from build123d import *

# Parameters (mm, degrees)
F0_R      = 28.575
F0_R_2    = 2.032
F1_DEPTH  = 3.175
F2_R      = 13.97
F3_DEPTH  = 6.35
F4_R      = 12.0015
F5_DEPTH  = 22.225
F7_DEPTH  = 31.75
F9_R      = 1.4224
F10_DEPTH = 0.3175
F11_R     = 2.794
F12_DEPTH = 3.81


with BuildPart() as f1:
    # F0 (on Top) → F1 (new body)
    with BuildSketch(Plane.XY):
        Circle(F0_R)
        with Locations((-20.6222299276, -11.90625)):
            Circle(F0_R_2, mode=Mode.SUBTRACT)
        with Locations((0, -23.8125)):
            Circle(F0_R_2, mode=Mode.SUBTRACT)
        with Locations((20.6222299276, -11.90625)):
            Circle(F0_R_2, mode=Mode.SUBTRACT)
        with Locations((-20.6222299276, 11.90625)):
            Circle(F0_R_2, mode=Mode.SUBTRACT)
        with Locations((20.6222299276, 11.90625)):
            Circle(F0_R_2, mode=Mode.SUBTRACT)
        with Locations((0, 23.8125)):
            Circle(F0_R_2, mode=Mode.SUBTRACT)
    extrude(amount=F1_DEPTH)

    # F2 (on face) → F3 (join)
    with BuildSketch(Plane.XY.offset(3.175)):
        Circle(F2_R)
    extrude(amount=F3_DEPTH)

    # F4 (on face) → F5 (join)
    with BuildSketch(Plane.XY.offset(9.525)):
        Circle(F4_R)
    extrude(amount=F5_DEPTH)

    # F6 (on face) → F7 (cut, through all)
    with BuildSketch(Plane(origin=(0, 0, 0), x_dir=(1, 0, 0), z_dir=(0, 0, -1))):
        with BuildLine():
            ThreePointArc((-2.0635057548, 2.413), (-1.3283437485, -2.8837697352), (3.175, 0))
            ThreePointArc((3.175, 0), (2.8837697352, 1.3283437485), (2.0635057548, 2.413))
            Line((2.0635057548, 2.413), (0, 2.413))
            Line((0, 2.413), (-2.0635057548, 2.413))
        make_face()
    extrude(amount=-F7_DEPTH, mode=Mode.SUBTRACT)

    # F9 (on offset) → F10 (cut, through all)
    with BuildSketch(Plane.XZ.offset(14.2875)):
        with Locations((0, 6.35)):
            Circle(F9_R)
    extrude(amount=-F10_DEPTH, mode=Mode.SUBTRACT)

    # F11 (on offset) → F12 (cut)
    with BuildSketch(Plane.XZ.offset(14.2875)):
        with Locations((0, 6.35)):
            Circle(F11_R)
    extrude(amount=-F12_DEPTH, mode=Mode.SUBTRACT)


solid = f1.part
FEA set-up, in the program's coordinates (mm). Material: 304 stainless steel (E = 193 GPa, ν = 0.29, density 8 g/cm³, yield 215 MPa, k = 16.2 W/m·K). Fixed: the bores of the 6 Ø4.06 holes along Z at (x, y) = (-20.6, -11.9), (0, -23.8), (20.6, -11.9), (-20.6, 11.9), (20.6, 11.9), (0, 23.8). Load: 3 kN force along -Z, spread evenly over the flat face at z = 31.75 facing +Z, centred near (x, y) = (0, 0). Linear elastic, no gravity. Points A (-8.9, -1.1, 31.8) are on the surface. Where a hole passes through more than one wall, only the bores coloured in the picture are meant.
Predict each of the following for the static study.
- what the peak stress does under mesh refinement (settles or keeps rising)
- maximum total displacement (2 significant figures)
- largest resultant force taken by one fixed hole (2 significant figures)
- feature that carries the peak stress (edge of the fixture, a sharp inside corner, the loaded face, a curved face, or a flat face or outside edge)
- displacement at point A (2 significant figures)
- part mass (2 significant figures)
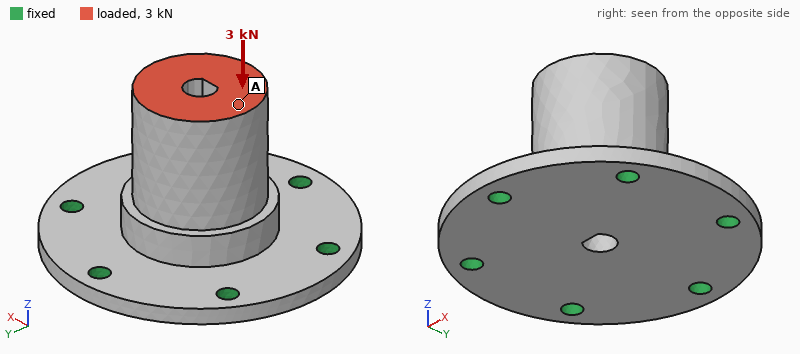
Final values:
keeps rising
10 µm
570 N
edge of the fixture
9.9 µm
170 g
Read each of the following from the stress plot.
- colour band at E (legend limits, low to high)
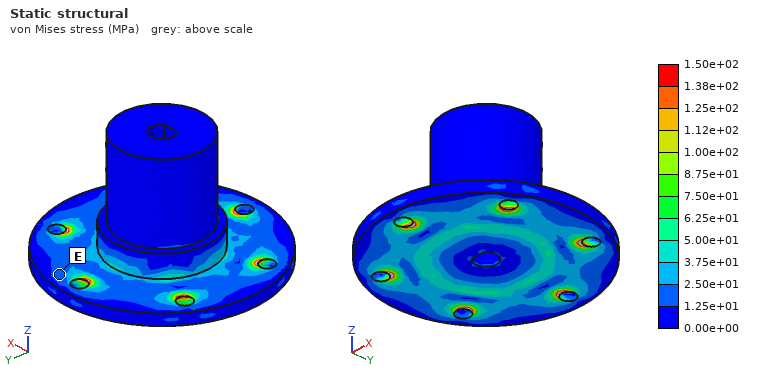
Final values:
1.25e+01 to 2.50e+01 MPa
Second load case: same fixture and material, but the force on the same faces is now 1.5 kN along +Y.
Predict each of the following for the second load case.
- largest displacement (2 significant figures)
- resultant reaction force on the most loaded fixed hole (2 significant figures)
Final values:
29 µm
890 N
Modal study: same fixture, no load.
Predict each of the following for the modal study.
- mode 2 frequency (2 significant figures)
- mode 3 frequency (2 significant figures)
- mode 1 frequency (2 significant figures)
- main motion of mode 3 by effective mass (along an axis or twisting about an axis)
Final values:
6200 Hz
8100 Hz
6100 Hz
along Z
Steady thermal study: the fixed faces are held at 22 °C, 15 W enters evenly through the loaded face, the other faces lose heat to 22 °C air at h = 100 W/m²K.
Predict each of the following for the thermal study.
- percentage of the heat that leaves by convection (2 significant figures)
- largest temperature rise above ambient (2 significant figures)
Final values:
72 %
54 K
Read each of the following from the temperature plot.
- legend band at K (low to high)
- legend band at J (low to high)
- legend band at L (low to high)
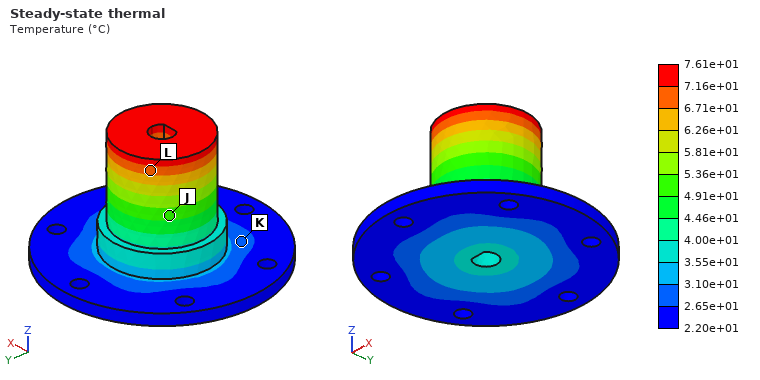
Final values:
2.65e+01 to 3.10e+01 °C
4.91e+01 to 5.36e+01 °C
6.71e+01 to 7.16e+01 °C
